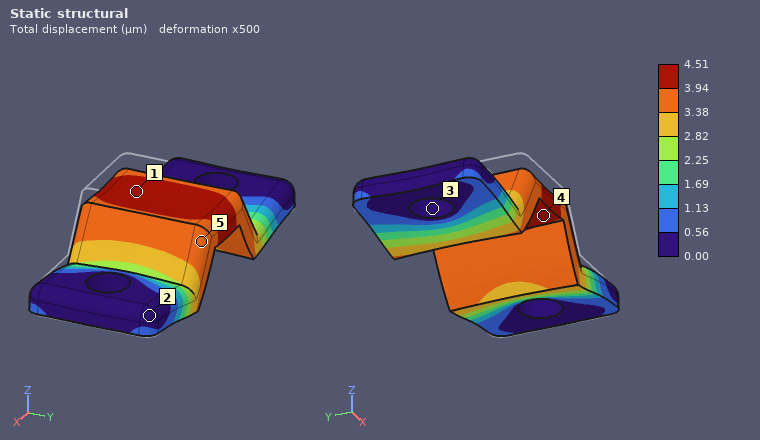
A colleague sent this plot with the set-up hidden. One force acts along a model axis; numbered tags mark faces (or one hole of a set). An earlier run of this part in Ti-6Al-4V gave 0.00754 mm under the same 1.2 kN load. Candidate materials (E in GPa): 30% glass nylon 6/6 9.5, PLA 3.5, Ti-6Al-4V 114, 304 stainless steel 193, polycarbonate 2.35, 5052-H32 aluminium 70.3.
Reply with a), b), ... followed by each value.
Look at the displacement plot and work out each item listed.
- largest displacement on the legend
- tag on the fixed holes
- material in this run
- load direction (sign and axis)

a) 4.51 µm
b) 3
c) 304 stainless steel
d) -Z
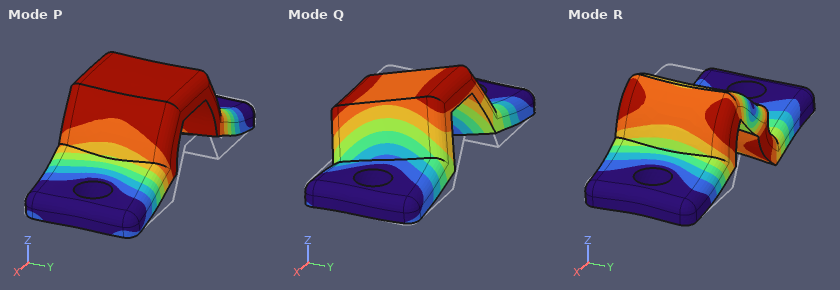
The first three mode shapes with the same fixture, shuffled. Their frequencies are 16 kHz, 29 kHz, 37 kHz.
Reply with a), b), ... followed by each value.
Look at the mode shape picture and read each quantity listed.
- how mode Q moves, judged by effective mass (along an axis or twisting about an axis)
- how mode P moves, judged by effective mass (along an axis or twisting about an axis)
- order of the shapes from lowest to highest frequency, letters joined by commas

a) along Y
b) along Z
c) Q, P, R
